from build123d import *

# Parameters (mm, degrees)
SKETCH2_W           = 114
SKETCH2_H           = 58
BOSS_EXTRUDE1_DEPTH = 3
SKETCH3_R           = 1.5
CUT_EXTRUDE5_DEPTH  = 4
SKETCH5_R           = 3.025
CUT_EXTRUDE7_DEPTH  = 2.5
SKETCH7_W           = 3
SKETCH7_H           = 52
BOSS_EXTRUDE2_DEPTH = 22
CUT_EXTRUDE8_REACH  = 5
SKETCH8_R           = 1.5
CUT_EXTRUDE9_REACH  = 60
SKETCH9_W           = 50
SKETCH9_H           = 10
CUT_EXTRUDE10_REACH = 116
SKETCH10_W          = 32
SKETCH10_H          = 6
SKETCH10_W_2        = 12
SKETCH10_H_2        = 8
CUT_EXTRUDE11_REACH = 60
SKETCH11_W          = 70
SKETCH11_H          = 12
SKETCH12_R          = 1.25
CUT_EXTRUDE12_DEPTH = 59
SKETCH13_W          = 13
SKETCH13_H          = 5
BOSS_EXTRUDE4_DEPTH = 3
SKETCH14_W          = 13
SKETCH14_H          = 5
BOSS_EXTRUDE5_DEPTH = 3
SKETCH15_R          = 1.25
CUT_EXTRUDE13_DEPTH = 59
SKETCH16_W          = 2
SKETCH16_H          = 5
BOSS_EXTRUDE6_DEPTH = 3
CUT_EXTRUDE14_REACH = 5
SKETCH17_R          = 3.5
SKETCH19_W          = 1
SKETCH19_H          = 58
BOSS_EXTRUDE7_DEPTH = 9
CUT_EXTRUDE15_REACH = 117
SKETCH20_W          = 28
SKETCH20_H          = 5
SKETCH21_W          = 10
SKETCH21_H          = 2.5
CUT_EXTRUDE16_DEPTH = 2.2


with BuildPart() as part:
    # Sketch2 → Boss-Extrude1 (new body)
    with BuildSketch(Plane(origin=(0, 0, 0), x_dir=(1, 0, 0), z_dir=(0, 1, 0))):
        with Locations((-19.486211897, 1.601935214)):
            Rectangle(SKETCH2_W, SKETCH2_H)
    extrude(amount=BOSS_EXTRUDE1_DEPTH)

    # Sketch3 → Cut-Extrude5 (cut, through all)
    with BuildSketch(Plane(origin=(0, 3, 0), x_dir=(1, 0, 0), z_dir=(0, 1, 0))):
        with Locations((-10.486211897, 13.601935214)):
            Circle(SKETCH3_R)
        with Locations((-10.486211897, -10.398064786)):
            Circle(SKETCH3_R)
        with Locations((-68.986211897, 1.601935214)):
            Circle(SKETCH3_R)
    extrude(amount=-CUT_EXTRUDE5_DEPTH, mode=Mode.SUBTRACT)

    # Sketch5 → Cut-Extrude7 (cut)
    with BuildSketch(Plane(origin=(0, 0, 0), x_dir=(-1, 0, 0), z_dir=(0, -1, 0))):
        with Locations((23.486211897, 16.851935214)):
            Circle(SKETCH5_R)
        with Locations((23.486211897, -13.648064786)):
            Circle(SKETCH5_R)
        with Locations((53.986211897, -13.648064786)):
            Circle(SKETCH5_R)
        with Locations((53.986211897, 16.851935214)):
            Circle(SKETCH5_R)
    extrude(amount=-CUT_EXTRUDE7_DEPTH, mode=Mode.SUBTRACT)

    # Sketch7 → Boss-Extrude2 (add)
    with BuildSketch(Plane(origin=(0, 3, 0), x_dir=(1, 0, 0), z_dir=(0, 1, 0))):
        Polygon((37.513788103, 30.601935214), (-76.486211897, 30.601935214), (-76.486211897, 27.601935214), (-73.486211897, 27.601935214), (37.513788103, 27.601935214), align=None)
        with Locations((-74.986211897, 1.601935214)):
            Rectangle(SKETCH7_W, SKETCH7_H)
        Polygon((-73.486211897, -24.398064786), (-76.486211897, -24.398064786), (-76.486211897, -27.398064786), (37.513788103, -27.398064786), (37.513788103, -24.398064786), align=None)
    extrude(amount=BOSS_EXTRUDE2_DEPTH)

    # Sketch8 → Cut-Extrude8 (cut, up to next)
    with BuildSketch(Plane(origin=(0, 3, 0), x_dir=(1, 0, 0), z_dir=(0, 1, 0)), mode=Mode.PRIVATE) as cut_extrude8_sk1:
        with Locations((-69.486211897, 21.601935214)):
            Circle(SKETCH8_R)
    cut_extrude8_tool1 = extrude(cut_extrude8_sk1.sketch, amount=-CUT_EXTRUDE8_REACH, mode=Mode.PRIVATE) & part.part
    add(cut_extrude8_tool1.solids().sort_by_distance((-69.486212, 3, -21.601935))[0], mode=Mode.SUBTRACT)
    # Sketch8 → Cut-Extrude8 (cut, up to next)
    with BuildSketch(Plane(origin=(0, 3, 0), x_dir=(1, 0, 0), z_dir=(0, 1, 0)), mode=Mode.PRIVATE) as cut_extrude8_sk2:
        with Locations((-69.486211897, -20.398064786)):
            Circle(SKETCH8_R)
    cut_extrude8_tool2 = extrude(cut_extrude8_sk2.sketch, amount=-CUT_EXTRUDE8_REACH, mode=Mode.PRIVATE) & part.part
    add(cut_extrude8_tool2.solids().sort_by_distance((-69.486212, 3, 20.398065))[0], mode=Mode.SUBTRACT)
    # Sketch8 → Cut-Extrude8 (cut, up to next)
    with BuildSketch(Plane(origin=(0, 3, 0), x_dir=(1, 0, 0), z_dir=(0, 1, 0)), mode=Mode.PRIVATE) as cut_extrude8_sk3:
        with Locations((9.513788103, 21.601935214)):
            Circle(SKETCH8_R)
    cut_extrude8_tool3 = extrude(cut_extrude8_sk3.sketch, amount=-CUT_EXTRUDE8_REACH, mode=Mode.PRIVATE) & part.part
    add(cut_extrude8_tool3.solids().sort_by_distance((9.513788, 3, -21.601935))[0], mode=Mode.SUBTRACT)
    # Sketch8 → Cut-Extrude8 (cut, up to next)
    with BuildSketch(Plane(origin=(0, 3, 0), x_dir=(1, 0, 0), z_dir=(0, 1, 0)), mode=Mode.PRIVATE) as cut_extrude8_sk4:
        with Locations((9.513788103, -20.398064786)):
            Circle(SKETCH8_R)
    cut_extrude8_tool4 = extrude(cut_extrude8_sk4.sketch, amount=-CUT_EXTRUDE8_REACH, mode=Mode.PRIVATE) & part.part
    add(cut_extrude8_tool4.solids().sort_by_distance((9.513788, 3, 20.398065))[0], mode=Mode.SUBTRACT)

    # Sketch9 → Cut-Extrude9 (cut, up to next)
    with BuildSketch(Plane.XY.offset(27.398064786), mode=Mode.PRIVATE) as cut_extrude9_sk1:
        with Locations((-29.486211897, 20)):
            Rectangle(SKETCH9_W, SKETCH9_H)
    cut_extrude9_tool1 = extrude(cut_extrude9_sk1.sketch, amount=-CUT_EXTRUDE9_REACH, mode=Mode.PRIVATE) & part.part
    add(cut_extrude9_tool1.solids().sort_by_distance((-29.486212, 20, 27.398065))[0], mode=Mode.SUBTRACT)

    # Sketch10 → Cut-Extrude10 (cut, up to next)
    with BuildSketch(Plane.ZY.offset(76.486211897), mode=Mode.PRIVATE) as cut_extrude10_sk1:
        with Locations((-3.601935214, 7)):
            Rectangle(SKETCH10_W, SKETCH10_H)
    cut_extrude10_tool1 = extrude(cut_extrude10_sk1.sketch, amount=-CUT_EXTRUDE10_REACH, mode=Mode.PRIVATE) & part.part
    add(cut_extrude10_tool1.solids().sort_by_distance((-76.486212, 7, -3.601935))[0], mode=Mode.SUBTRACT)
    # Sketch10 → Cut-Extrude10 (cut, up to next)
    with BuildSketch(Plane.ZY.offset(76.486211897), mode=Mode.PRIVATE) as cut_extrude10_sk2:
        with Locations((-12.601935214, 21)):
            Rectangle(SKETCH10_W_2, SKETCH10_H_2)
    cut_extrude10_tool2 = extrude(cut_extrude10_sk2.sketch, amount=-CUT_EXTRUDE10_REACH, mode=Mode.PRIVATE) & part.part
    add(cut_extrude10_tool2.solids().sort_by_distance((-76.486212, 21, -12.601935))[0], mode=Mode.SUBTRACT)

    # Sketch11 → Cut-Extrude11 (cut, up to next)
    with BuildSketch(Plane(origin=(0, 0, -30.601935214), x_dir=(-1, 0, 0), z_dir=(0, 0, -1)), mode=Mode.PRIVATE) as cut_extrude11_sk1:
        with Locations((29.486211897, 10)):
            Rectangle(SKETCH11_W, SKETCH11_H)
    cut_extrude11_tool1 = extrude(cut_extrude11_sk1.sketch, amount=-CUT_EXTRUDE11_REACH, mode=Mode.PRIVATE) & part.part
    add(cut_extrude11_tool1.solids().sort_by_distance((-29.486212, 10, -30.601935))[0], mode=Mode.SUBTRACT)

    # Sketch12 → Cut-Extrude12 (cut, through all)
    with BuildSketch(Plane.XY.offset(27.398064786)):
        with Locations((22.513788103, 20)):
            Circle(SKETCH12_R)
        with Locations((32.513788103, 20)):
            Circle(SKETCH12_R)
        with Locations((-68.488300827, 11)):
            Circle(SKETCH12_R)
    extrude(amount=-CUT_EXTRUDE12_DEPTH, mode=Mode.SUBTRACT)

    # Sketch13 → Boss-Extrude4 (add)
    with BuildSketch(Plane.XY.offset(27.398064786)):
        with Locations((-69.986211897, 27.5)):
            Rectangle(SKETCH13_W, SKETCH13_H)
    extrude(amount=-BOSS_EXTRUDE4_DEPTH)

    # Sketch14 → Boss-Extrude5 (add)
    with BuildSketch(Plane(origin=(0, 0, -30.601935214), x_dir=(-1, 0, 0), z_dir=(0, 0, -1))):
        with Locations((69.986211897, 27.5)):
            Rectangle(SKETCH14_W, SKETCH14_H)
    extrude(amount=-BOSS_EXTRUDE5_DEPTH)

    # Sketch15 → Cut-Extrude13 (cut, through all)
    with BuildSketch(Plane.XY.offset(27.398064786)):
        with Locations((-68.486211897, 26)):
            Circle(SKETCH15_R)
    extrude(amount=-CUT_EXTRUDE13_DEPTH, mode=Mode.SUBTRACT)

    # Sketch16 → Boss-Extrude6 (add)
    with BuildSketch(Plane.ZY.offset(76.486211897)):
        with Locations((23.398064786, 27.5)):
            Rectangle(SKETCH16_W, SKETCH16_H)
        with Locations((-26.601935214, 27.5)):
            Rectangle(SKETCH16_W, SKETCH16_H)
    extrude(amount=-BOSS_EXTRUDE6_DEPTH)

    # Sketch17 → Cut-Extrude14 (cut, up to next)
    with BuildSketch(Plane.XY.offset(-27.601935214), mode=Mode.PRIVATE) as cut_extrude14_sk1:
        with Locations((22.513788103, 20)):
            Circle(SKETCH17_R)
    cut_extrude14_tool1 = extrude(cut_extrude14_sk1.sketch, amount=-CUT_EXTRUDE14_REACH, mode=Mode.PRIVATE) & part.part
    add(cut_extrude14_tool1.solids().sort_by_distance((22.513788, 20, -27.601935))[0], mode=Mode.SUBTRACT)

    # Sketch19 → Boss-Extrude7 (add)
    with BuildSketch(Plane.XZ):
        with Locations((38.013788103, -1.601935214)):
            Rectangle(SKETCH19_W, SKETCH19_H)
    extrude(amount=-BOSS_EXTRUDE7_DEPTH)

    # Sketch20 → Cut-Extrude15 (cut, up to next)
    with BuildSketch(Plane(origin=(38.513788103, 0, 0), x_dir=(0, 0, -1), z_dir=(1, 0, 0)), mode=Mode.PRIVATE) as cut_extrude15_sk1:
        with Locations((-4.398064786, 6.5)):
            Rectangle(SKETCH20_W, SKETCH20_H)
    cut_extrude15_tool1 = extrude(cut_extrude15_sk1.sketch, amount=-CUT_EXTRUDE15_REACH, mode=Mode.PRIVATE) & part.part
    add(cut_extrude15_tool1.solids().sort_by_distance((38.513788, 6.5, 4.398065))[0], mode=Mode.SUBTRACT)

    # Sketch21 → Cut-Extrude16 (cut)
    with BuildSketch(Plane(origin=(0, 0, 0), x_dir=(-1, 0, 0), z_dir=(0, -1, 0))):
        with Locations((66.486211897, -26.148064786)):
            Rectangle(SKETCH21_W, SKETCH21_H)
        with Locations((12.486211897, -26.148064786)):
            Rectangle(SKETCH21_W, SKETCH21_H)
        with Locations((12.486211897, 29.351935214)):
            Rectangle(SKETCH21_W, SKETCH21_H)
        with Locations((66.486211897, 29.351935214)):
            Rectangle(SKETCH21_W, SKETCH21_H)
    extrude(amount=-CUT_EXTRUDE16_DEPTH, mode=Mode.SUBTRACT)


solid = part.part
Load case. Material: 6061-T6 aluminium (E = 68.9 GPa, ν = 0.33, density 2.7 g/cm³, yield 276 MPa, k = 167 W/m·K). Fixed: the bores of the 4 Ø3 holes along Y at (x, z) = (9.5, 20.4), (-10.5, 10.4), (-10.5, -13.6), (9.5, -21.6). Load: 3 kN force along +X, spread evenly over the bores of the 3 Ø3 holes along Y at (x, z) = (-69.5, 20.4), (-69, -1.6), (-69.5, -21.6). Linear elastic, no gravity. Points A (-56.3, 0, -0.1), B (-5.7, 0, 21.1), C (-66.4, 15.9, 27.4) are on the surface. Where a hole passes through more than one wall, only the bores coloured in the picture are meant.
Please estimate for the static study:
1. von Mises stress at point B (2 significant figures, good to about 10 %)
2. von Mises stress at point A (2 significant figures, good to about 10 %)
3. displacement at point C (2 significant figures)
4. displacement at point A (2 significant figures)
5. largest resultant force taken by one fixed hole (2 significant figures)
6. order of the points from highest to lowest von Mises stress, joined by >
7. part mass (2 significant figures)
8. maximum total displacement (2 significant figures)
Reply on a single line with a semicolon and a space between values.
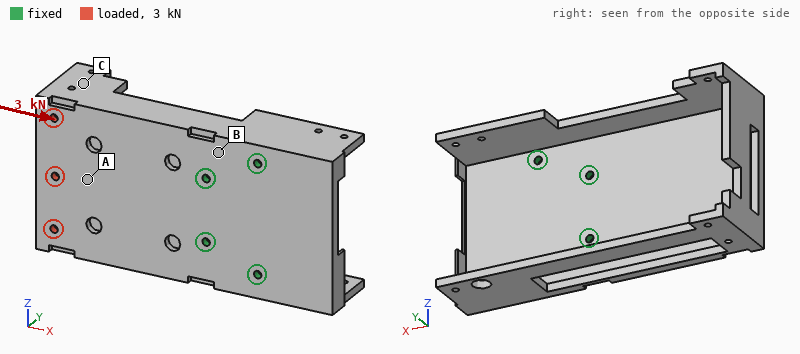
13 MPa; 21 MPa; 40 µm; 29 µm; 1.1 kN; A > B > C; 90 g; 58 µm
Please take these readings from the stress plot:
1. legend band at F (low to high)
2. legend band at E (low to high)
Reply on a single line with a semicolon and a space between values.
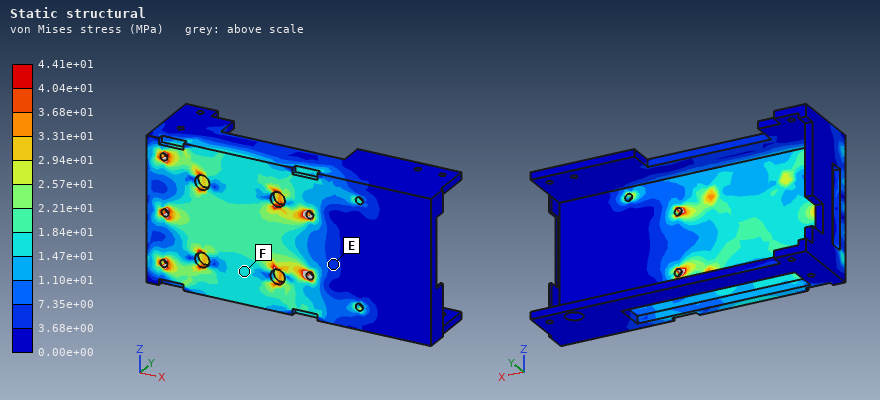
1.47e+01 to 1.84e+01 MPa; 3.68e+00 to 7.35e+00 MPa
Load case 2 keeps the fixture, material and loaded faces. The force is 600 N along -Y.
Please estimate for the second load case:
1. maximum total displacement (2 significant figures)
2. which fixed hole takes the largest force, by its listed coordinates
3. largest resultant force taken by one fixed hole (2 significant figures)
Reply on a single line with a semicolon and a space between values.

1.2 mm; (-10.5, 10.4); 1.2 kN
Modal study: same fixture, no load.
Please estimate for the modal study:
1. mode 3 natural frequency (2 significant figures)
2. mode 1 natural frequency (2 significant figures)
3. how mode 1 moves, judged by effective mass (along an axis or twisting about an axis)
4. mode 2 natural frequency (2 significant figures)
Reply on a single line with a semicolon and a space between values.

1800 Hz; 720 Hz; along Y; 950 Hz
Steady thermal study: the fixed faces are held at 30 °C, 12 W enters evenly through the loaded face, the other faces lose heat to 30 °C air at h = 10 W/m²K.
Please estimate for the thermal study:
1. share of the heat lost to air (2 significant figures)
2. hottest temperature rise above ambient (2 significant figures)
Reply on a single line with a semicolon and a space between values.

16 %; 21 K
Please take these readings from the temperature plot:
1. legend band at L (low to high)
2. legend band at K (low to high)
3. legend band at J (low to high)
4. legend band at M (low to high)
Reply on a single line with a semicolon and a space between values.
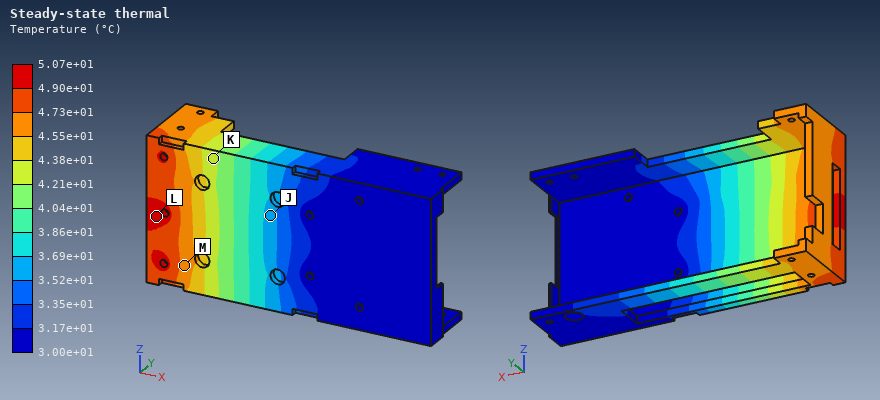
4.90e+01 to 5.07e+01 °C; 4.21e+01 to 4.38e+01 °C; 3.52e+01 to 3.69e+01 °C; 4.55e+01 to 4.73e+01 °C
